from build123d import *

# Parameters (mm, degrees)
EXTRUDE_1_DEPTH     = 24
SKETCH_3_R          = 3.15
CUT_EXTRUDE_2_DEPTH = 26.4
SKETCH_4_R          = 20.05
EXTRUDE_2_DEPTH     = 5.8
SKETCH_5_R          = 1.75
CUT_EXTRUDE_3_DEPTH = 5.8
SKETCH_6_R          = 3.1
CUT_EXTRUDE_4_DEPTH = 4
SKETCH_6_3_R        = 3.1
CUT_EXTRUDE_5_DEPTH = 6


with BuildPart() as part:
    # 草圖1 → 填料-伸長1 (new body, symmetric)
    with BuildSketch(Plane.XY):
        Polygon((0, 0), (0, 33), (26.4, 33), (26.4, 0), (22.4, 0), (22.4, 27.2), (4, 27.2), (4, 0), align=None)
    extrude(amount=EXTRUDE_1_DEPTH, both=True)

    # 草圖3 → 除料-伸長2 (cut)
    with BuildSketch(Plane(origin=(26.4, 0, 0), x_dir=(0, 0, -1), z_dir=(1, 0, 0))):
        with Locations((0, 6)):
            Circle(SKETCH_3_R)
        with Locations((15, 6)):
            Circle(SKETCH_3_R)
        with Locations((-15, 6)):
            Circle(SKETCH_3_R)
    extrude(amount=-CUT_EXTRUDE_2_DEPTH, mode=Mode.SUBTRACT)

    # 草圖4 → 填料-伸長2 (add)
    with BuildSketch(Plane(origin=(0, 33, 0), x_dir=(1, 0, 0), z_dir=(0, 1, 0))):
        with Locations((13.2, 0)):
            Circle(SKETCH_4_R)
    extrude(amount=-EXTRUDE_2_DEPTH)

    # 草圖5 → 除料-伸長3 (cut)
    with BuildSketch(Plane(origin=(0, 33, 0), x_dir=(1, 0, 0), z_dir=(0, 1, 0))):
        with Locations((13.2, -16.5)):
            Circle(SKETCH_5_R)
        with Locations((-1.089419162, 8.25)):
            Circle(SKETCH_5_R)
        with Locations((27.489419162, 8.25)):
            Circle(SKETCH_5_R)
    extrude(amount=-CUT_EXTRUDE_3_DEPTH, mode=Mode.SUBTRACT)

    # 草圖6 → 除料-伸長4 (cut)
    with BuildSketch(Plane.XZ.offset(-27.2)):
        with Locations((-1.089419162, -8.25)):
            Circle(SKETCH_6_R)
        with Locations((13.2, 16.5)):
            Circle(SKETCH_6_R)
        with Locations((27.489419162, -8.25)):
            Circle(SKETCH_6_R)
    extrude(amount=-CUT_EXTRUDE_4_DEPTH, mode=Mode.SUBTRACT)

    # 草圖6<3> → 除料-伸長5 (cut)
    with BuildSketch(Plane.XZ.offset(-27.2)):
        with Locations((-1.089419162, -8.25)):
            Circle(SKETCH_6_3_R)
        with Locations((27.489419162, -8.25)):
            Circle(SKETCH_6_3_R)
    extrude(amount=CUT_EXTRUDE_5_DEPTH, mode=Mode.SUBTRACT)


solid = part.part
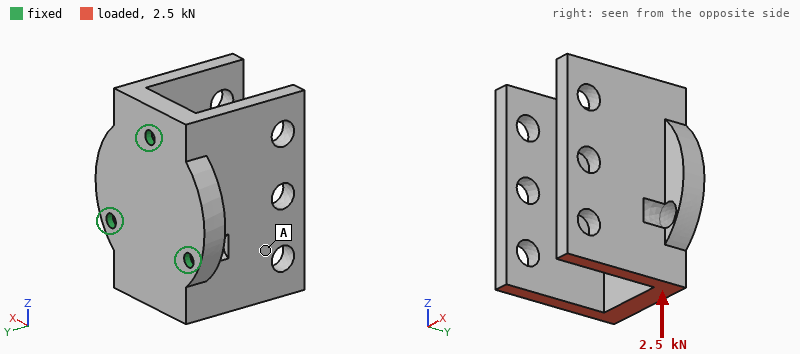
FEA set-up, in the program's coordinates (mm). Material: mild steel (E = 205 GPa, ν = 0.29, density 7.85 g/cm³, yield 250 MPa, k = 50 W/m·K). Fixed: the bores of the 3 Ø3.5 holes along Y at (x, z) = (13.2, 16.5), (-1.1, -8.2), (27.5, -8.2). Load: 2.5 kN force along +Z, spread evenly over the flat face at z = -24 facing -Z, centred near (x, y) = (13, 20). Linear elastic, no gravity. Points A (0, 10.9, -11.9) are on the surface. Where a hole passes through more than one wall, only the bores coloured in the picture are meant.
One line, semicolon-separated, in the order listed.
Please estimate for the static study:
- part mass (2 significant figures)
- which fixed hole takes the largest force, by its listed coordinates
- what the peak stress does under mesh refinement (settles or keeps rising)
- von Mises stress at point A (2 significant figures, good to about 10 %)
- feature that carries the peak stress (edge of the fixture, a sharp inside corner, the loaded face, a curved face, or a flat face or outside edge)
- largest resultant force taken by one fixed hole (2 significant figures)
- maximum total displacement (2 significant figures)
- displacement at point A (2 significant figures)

140 g; (13.2, 16.5); keeps rising; 13 MPa; edge of the fixture; 1.4 kN; 18 µm; 9.9 µm
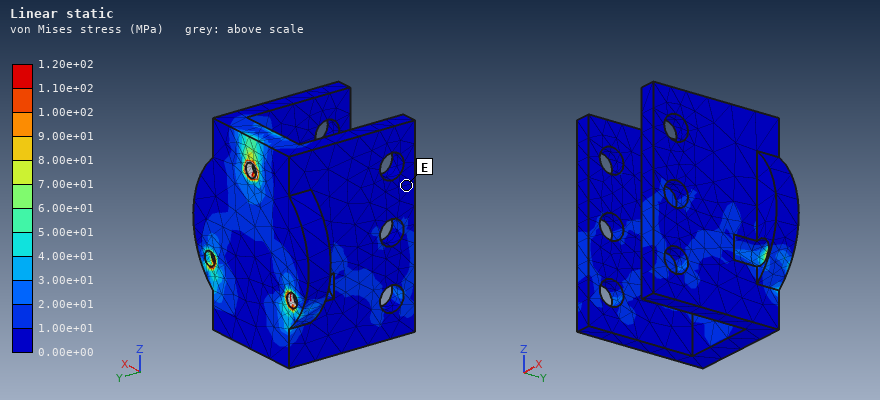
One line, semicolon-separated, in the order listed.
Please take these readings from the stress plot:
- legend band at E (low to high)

0.00e+00 to 1.00e+01 MPa
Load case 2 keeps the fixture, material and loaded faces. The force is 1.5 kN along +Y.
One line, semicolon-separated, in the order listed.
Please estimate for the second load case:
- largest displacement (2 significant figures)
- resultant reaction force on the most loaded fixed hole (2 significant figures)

20 µm; 1.3 kN
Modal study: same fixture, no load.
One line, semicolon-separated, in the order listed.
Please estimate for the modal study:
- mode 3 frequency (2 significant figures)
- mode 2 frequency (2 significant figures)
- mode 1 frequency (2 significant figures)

5600 Hz; 3600 Hz; 3500 Hz
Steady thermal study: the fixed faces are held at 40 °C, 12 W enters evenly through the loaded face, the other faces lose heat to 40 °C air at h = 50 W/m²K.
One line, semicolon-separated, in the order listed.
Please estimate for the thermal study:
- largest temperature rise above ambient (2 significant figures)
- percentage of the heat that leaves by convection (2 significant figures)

22 K; 33 %
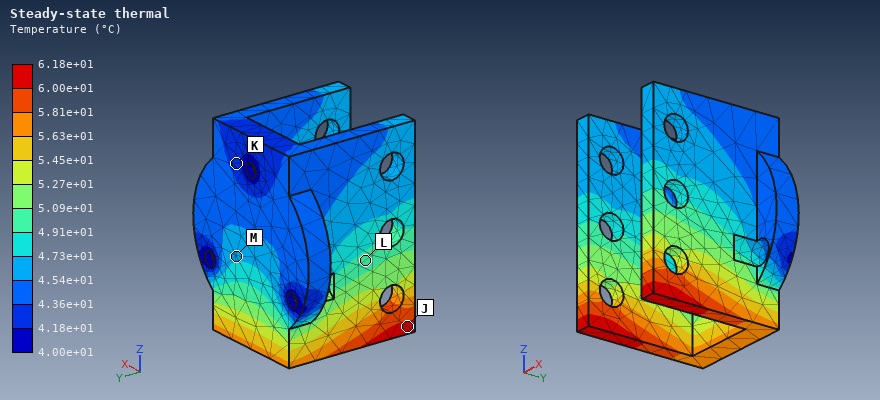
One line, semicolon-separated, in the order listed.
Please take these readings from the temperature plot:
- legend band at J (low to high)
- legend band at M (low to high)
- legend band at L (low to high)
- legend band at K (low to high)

6.00e+01 to 6.18e+01 °C; 4.54e+01 to 4.73e+01 °C; 4.91e+01 to 5.09e+01 °C; 4.18e+01 to 4.36e+01 °C
